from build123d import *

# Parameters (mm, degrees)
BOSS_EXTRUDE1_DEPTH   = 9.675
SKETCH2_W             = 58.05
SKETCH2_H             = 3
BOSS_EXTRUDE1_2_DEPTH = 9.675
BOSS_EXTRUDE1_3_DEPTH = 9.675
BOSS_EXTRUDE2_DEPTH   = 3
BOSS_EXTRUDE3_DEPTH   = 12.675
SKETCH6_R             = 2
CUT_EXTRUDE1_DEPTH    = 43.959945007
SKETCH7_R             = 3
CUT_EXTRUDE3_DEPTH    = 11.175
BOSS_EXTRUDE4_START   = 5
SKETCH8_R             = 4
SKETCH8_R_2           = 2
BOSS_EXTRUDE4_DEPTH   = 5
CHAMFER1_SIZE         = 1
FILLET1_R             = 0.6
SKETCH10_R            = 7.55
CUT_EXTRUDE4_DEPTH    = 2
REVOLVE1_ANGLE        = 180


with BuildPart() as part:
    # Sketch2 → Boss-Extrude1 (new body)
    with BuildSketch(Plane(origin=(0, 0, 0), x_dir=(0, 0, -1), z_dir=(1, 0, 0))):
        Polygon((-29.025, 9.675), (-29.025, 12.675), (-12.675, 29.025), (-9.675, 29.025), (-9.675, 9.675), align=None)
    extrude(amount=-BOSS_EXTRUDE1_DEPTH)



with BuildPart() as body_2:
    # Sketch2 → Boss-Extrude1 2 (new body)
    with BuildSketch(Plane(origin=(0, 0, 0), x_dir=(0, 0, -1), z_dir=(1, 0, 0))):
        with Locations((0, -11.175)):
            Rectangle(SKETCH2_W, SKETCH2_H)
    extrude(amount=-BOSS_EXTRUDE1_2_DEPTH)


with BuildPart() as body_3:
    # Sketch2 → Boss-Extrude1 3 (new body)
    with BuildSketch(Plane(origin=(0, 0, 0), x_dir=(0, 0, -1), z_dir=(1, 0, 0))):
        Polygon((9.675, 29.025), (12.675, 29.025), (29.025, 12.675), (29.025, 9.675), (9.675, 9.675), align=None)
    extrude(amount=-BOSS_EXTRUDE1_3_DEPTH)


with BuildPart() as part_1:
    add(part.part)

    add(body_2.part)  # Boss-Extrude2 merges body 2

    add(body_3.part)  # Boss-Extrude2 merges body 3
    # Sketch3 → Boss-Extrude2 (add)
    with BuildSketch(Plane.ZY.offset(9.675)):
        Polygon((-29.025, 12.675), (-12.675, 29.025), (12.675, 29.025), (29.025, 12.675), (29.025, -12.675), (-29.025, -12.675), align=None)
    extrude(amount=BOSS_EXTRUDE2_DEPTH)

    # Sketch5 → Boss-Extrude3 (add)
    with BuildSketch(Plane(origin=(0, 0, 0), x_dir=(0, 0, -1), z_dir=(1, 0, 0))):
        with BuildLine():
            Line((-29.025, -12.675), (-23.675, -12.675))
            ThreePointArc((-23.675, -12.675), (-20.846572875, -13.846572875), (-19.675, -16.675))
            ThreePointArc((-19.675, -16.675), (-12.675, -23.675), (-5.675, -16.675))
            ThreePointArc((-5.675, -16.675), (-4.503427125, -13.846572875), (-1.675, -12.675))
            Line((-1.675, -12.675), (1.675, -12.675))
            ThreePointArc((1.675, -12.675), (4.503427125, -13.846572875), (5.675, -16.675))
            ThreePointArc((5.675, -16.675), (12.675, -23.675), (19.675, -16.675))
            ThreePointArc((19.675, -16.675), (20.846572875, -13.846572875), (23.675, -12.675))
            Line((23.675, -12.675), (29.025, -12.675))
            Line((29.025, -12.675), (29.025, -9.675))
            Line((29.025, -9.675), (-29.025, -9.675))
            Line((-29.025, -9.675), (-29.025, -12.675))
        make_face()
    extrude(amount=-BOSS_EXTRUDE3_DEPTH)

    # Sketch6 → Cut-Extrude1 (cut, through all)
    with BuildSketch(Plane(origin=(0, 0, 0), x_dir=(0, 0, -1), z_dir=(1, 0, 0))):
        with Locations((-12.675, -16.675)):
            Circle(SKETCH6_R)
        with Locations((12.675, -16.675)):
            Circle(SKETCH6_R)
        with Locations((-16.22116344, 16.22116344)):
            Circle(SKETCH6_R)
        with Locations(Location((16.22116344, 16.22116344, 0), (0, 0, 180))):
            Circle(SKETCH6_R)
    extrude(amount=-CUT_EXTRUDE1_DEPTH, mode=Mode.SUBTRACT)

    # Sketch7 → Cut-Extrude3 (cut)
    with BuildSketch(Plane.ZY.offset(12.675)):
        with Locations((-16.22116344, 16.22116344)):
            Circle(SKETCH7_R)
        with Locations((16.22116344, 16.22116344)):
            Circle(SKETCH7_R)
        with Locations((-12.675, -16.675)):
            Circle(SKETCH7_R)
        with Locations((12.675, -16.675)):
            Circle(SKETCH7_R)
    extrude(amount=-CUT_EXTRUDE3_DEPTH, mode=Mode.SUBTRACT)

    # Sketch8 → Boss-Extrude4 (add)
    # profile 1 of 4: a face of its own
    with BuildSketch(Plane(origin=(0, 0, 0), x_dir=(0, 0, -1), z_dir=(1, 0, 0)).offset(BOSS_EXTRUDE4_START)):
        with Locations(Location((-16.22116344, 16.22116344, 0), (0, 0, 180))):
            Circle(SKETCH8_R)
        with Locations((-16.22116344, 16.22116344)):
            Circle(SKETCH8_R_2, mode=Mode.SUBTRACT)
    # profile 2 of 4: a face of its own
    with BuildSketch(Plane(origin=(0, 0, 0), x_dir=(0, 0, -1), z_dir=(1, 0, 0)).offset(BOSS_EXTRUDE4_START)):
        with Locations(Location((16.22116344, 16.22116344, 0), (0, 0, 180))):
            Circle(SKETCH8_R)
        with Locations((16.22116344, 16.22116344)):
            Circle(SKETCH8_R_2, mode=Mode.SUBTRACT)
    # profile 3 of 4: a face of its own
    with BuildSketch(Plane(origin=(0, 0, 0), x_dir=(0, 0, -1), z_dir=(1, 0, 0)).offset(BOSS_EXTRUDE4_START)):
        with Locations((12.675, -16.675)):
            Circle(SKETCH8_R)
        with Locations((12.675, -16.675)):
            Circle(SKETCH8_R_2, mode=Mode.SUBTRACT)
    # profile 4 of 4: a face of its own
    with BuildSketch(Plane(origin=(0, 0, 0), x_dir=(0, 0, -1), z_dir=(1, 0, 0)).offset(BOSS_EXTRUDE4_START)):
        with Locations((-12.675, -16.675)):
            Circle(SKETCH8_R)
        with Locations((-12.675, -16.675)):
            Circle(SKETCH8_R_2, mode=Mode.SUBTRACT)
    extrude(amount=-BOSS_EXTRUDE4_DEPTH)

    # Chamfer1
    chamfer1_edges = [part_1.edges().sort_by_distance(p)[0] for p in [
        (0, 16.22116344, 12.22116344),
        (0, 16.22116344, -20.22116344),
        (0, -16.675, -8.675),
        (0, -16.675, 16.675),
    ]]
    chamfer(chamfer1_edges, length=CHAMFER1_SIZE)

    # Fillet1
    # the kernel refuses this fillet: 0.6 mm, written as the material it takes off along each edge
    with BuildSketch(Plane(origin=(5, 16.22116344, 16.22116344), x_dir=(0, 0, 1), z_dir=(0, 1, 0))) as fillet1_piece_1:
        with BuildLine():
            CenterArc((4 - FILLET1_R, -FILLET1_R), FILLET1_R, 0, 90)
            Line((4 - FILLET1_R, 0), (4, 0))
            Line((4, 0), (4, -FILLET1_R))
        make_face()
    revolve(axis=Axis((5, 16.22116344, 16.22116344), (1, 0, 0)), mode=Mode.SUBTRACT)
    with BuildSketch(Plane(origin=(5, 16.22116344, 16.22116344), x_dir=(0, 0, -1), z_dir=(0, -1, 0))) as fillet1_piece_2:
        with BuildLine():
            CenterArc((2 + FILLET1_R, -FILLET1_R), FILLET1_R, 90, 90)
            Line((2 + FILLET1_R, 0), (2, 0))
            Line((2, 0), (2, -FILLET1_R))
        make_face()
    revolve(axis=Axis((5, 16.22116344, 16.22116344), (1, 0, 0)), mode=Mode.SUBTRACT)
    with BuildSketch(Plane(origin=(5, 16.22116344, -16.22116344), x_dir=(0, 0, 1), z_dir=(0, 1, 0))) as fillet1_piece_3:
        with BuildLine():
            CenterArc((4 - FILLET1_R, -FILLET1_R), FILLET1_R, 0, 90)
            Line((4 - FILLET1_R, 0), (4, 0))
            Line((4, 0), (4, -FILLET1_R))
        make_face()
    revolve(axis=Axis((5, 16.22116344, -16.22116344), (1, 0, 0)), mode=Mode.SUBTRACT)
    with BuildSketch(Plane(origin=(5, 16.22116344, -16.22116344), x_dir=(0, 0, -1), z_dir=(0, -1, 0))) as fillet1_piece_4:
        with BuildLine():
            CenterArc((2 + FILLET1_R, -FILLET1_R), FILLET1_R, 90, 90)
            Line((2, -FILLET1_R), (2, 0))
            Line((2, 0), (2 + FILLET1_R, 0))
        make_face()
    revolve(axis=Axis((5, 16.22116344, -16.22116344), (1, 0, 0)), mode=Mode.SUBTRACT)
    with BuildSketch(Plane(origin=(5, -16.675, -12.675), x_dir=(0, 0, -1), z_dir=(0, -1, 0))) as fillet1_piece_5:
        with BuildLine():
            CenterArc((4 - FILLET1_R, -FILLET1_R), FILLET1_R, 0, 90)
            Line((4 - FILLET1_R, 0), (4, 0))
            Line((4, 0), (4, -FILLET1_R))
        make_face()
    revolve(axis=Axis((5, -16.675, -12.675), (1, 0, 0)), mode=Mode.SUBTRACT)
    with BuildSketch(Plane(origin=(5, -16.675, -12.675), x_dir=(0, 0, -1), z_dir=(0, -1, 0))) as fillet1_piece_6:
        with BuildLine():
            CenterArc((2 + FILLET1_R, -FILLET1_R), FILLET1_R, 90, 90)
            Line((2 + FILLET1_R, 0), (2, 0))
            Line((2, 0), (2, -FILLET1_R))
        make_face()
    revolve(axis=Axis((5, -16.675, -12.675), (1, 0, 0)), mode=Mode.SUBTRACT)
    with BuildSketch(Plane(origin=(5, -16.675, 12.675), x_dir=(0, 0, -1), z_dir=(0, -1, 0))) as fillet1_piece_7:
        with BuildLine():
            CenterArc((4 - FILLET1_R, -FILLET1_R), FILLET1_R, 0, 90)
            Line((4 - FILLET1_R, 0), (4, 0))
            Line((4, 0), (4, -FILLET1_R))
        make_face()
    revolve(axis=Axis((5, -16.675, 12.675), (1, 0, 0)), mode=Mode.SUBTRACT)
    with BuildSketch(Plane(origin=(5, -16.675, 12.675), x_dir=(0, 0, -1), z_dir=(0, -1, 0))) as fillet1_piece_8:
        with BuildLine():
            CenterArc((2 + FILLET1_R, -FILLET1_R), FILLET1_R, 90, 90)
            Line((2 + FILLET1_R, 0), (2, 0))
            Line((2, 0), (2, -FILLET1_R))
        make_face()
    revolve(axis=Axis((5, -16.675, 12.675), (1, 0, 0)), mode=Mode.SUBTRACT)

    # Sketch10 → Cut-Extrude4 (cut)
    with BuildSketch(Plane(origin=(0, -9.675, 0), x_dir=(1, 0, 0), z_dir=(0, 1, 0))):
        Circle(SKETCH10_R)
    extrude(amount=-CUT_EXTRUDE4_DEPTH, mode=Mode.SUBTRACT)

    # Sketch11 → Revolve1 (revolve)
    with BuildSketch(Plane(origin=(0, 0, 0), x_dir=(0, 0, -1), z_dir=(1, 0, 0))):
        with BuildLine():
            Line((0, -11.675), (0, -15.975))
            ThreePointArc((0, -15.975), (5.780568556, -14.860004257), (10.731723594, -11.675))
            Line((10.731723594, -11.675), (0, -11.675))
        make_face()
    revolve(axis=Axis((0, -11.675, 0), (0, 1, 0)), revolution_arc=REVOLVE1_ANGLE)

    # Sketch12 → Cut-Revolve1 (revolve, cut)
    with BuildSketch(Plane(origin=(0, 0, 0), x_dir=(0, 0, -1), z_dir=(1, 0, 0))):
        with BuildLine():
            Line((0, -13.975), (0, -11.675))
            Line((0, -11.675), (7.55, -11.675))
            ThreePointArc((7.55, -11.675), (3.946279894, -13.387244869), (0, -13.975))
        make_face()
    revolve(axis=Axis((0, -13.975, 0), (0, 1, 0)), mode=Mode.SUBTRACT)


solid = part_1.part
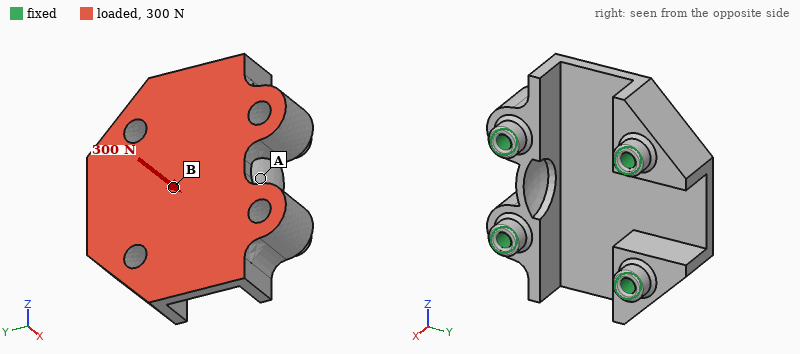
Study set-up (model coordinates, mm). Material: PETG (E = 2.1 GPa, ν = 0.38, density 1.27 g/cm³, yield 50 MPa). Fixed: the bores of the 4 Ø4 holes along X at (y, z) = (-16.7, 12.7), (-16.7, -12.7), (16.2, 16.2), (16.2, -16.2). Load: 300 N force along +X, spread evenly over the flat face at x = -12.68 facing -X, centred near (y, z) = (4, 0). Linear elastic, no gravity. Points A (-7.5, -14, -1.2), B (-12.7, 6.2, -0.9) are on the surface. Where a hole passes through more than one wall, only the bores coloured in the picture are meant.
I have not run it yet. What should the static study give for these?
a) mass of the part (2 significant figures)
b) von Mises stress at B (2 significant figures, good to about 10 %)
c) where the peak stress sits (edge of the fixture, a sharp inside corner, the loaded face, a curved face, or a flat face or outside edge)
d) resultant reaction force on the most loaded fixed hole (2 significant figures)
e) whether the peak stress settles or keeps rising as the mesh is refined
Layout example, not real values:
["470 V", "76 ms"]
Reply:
["20 g", "1.8 MPa", "edge of the fixture", "94 N", "keeps rising"]
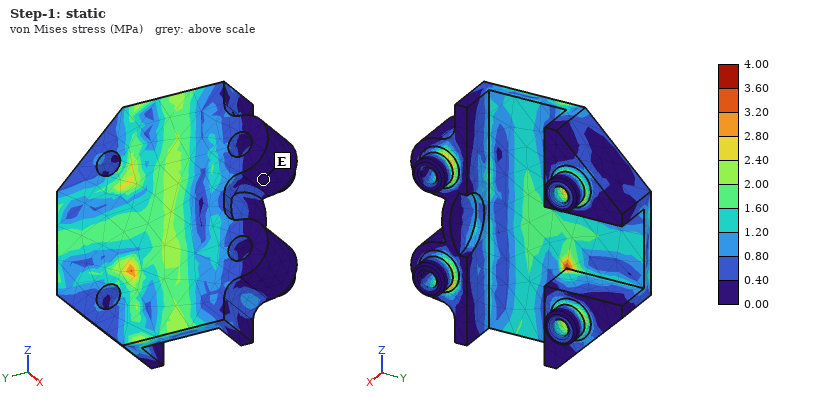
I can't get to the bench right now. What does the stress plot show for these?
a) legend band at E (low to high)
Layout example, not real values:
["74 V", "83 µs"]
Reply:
["0.00 to 0.40 MPa"]
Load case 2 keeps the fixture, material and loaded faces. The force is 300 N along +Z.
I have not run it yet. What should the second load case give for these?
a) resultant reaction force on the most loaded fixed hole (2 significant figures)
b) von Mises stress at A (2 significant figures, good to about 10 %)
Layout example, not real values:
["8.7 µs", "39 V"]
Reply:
["110 N", "3.7 MPa"]
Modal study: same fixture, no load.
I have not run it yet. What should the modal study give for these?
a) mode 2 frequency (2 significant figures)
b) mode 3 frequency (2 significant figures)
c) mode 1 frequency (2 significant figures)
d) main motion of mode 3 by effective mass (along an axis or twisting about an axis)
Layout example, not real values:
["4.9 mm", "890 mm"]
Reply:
["2900 Hz", "3700 Hz", "2900 Hz", "along Z"]
